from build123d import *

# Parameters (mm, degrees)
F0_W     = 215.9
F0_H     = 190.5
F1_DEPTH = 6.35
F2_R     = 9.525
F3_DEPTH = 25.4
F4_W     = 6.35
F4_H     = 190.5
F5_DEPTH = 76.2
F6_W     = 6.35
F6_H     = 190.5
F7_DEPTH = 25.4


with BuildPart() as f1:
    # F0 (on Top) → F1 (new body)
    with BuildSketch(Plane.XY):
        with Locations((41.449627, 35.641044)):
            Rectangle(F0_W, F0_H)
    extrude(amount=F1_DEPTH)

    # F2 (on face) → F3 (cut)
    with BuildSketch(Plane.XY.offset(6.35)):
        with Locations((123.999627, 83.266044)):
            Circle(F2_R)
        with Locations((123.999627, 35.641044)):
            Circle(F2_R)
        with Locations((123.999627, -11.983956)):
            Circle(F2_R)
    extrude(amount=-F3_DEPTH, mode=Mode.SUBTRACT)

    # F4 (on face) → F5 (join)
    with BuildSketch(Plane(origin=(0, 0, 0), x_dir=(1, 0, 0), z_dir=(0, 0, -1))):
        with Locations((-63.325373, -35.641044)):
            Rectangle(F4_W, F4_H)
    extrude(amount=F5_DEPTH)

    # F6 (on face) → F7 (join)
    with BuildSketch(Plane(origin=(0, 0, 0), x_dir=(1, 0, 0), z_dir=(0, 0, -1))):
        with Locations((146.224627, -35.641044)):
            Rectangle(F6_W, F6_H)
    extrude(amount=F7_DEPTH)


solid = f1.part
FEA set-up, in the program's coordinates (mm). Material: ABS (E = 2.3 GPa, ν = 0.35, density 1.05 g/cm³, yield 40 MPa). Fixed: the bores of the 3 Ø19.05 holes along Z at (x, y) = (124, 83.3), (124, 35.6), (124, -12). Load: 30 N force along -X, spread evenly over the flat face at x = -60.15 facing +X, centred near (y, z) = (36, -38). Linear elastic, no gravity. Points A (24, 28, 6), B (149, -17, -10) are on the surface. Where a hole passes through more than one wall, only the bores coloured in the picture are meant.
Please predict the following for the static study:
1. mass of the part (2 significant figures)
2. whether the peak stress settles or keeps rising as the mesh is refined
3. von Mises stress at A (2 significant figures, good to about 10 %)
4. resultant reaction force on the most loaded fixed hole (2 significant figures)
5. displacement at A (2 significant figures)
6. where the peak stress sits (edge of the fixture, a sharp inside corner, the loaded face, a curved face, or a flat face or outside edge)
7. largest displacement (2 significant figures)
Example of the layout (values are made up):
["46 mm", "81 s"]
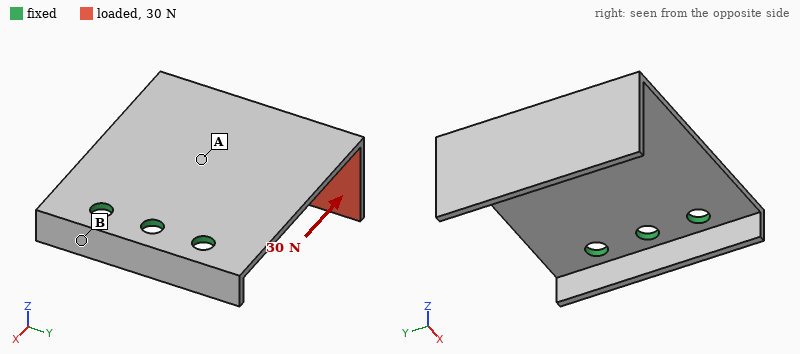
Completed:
["400 g", "keeps rising", "0.82 MPa", "12 N", "0.56 mm", "edge of the fixture", "2.9 mm"]
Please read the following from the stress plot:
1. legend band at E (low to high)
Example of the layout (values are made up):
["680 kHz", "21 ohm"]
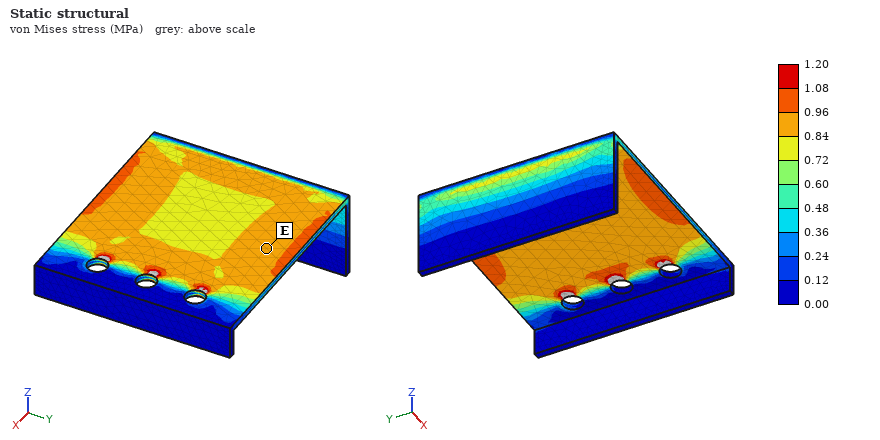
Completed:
["0.84 to 0.96 MPa"]
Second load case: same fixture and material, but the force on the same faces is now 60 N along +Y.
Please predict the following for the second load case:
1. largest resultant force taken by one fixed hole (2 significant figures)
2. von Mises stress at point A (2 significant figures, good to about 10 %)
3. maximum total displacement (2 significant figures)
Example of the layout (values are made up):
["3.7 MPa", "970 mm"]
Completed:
["100 N", "1.3 MPa", "2.8 mm"]
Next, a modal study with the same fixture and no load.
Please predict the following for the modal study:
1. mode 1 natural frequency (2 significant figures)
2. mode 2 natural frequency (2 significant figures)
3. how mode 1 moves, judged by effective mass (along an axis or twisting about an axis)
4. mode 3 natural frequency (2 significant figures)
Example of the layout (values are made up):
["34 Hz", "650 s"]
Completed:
["27 Hz", "62 Hz", "along Z", "130 Hz"]
